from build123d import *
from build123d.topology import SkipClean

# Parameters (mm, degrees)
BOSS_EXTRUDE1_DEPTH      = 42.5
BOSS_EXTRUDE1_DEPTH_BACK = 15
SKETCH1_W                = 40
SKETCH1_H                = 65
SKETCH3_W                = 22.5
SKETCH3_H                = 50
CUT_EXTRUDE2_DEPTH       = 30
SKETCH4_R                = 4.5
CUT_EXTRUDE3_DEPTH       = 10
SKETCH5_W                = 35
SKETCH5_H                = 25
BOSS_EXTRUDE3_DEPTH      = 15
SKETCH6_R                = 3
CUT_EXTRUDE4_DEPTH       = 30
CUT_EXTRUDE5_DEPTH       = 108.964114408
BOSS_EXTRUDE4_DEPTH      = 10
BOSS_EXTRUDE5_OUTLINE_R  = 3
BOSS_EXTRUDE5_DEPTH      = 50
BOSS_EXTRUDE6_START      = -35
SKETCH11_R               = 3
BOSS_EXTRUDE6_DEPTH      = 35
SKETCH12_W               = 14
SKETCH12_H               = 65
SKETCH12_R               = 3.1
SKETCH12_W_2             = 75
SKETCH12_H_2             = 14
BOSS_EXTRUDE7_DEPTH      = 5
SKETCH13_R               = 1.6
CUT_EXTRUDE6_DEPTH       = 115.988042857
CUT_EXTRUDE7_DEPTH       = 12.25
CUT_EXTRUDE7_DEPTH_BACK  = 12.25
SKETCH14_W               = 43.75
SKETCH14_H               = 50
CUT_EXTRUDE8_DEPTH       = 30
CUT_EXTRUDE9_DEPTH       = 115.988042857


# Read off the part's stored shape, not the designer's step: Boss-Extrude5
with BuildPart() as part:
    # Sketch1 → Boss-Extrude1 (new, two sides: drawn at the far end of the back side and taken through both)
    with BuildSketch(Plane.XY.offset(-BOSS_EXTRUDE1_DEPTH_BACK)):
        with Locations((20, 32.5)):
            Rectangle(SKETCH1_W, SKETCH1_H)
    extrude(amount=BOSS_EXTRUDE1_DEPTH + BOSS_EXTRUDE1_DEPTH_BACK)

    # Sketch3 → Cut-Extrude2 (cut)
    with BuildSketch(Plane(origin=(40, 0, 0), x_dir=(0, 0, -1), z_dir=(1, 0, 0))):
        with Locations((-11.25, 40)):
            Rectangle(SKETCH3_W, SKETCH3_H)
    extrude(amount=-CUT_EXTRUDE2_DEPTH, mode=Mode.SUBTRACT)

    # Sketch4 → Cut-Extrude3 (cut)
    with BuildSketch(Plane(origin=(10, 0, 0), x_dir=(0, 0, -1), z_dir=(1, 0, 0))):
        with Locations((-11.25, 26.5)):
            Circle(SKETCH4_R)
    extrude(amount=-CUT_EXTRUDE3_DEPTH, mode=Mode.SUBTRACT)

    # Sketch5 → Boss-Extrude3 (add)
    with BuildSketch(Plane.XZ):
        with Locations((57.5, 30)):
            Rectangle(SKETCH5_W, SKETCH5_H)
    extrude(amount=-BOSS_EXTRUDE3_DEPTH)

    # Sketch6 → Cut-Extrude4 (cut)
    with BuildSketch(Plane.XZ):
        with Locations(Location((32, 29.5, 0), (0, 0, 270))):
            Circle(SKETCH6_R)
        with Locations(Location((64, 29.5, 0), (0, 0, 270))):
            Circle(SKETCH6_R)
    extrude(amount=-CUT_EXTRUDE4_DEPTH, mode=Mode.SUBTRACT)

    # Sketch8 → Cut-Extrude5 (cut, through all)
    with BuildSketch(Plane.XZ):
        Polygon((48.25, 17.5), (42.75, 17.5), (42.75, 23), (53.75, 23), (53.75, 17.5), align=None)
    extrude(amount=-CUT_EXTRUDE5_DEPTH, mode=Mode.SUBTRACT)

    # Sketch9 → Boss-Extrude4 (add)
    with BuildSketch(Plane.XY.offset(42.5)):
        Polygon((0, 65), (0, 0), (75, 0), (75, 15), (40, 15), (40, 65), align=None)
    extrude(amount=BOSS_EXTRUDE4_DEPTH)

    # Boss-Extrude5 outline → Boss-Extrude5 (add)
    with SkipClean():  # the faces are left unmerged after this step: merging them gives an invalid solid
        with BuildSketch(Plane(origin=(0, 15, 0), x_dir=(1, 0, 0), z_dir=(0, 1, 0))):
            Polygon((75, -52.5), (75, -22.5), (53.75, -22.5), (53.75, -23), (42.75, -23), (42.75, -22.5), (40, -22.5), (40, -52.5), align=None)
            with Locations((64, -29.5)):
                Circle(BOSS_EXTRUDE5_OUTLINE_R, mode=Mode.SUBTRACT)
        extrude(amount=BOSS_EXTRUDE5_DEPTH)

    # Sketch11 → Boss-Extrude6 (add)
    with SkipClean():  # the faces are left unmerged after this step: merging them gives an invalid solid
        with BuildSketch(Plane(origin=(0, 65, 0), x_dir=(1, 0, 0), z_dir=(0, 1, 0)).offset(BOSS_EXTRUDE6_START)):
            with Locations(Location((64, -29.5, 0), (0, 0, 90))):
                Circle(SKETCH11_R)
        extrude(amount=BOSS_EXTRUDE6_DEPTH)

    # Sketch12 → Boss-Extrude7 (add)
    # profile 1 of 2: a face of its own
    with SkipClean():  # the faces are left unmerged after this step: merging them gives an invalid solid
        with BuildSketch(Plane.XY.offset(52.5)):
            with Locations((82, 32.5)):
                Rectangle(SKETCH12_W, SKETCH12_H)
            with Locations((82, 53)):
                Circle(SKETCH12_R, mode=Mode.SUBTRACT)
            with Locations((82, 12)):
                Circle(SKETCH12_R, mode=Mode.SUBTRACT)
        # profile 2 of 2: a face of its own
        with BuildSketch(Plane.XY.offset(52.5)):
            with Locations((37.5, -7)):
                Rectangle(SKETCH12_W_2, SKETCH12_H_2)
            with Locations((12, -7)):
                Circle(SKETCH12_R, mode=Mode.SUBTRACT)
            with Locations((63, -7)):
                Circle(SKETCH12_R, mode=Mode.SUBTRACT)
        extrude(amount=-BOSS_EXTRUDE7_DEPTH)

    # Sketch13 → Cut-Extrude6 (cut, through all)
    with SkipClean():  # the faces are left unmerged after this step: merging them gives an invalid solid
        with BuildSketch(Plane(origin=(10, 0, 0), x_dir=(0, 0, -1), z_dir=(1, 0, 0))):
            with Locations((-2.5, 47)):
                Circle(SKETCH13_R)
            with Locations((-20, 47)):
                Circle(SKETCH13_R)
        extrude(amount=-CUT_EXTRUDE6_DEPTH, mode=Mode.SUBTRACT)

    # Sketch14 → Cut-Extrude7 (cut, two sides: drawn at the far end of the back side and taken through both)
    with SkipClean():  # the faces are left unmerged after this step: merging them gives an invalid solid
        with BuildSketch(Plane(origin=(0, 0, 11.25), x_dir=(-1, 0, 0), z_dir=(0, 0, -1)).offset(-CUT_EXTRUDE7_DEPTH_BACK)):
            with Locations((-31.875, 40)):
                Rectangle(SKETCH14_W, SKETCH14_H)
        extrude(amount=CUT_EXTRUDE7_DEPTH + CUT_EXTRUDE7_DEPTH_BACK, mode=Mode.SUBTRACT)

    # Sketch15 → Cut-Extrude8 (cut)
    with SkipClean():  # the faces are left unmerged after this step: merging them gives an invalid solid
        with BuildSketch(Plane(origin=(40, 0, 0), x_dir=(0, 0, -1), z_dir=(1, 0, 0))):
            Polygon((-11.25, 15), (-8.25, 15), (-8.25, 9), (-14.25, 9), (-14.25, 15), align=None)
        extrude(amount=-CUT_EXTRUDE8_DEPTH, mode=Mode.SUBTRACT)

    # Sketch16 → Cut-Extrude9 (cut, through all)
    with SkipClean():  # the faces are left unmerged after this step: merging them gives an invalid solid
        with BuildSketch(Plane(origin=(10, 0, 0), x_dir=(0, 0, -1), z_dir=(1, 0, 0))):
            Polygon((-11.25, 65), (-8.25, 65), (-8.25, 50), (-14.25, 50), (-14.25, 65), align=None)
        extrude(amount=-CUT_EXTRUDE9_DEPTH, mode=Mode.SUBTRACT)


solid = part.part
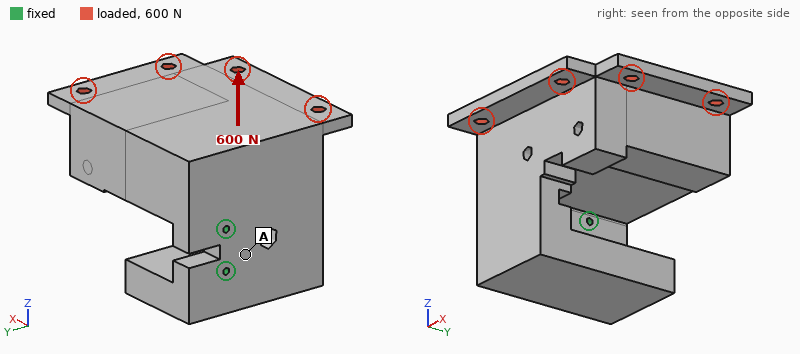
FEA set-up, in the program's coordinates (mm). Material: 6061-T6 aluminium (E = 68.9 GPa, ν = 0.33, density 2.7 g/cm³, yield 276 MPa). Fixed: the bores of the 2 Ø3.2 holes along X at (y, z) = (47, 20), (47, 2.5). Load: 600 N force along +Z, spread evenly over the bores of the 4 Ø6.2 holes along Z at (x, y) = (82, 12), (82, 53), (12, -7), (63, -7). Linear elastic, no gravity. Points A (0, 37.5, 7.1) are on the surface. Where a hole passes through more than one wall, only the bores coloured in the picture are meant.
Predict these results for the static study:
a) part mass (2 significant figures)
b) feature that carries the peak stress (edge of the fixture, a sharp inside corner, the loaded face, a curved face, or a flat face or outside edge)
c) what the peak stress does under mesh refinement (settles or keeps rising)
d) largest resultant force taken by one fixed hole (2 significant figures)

570 g
edge of the fixture
keeps rising
1.4 kN
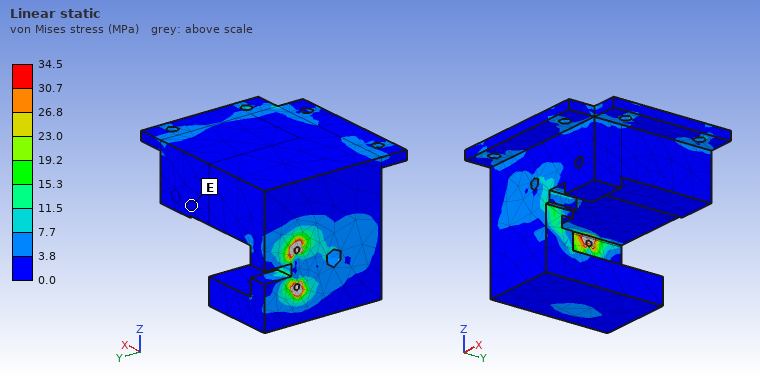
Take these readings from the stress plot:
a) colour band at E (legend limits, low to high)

0.0 to 3.8 MPa
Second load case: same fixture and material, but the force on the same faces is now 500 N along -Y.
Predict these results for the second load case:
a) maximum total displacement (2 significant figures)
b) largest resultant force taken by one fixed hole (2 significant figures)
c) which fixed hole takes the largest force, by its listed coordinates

94 µm
1.2 kN
(47, 20)
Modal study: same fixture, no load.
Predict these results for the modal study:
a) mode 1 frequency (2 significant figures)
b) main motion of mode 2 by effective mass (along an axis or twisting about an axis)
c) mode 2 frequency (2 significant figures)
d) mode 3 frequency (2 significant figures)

800 Hz
along Z
1000 Hz
2300 Hz
